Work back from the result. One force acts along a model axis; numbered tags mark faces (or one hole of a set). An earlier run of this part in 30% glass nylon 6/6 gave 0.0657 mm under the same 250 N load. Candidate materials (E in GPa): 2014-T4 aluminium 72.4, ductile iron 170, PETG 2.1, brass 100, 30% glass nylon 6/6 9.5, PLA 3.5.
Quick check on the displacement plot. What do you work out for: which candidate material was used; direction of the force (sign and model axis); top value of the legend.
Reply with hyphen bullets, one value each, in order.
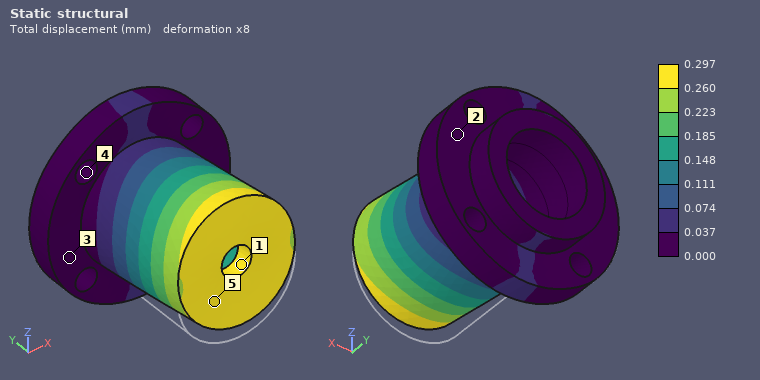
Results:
- PETG
- +Z
- 0.297 mm
